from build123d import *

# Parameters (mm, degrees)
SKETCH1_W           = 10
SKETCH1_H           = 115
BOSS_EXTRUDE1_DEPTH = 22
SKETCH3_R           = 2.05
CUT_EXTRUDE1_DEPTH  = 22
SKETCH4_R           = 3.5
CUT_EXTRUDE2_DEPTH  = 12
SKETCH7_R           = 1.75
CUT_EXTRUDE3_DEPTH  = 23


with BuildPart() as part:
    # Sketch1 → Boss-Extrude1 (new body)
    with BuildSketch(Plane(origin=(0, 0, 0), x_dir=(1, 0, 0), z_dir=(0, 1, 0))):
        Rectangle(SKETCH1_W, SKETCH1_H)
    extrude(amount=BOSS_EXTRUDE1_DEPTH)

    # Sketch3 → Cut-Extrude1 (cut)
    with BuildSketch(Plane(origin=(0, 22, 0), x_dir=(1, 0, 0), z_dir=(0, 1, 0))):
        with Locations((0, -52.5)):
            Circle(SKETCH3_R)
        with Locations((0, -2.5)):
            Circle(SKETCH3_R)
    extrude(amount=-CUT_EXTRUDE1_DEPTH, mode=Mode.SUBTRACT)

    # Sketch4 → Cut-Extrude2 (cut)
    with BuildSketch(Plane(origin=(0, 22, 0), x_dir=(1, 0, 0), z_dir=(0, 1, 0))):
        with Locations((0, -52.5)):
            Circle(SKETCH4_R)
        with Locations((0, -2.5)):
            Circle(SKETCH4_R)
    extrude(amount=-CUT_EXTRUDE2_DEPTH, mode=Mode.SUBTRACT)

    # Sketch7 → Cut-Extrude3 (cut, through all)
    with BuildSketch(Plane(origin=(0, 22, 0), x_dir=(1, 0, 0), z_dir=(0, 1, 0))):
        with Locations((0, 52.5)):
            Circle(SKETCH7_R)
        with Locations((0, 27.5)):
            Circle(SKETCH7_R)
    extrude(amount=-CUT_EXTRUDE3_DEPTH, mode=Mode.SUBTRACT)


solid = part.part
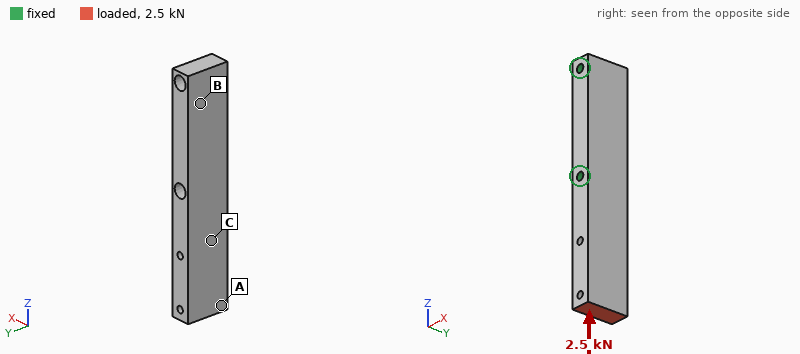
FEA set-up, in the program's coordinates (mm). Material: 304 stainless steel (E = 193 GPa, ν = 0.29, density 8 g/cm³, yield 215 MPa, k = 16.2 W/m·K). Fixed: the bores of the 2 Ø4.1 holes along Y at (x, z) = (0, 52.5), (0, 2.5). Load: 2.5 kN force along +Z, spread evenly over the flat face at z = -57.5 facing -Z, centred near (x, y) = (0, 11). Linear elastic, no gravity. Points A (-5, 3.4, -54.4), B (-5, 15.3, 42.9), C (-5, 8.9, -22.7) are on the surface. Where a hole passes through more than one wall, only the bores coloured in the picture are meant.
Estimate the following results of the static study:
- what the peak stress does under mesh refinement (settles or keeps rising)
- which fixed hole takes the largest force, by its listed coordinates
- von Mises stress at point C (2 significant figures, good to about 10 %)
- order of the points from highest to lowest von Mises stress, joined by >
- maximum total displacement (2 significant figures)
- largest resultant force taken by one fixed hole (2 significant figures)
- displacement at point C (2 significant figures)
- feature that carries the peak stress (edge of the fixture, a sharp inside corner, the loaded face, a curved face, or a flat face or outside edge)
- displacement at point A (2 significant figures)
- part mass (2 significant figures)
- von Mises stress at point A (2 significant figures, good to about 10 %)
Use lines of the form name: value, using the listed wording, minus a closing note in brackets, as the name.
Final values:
what the peak stress does under mesh refinement: keeps rising
which fixed hole takes the largest force, by its listed coordinates: (0, 2.5)
von Mises stress at point C: 15 MPa
order of the points from highest to lowest von Mises stress, joined by >: C > A > B
maximum total displacement: 11 µm
largest resultant force taken by one fixed hole: 2.1 kN
displacement at point C: 4.0 µm
feature that carries the peak stress: edge of the fixture
displacement at point A: 8.4 µm
part mass: 190 g
von Mises stress at point A: 11 MPa
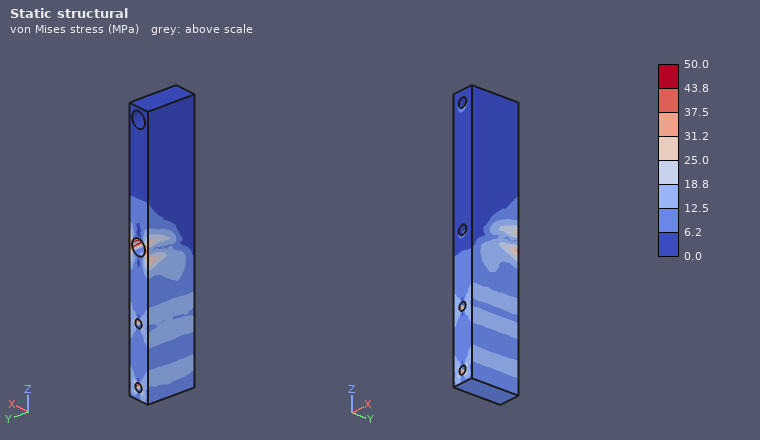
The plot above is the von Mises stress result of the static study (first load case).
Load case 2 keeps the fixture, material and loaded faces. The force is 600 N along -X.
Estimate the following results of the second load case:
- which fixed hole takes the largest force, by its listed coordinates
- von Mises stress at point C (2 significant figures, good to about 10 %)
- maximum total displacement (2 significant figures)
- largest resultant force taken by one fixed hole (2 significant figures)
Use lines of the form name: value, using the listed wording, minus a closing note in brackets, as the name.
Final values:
which fixed hole takes the largest force, by its listed coordinates: (0, 2.5)
von Mises stress at point C: 59 MPa
maximum total displacement: 0.16 mm
largest resultant force taken by one fixed hole: 920 N
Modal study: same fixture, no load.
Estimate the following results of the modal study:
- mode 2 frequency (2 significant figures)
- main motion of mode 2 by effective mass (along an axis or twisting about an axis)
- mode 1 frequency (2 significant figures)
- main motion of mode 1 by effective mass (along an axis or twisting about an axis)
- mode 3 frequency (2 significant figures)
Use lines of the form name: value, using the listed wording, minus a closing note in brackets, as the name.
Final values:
mode 2 frequency: 3400 Hz
main motion of mode 2 by effective mass: along Y
mode 1 frequency: 1900 Hz
main motion of mode 1 by effective mass: along X
mode 3 frequency: 7800 Hz
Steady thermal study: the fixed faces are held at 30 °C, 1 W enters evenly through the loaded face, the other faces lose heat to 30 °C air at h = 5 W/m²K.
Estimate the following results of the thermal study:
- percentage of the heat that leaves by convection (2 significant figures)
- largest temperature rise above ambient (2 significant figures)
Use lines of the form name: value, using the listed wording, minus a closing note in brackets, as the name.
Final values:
percentage of the heat that leaves by convection: 19 %
largest temperature rise above ambient: 17 K
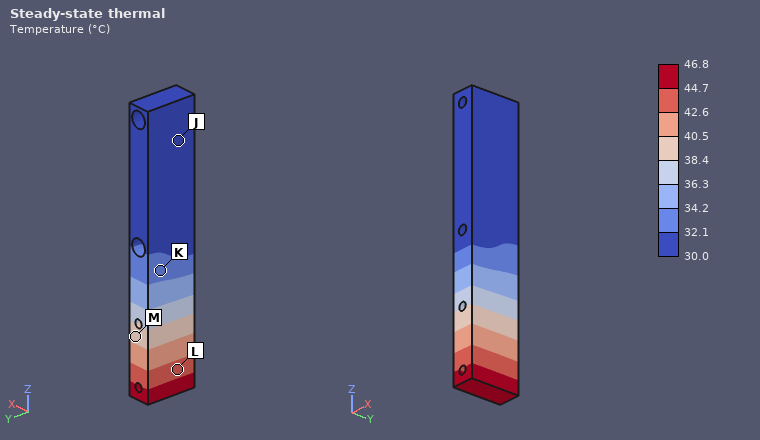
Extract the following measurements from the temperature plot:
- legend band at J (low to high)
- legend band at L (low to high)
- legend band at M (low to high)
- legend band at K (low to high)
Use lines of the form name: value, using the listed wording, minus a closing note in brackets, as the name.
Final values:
legend band at J: 30.0 to 32.1 °C
legend band at L: 42.6 to 44.7 °C
legend band at M: 38.4 to 40.5 °C
legend band at K: 32.1 to 34.2 °C
